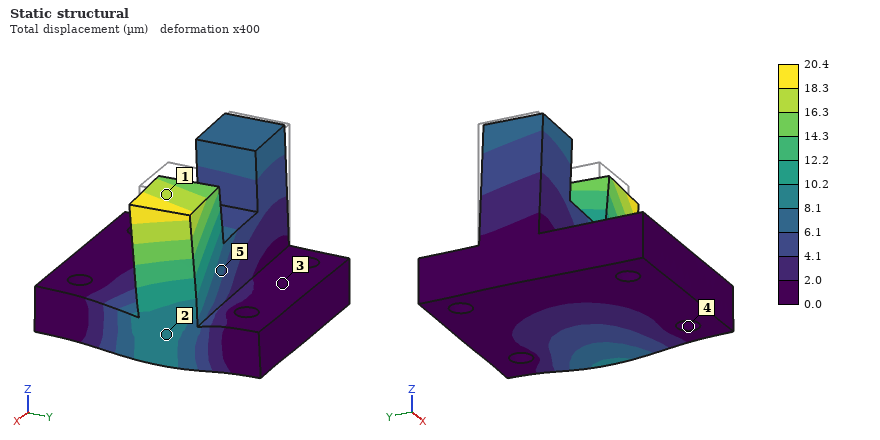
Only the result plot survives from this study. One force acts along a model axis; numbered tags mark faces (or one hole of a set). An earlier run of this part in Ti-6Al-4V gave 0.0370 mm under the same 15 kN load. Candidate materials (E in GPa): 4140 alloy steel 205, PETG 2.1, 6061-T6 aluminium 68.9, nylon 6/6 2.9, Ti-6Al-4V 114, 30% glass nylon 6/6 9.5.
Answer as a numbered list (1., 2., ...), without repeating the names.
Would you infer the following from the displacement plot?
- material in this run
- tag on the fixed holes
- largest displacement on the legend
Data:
1. 4140 alloy steel
2. 4
3. 20.4 µm
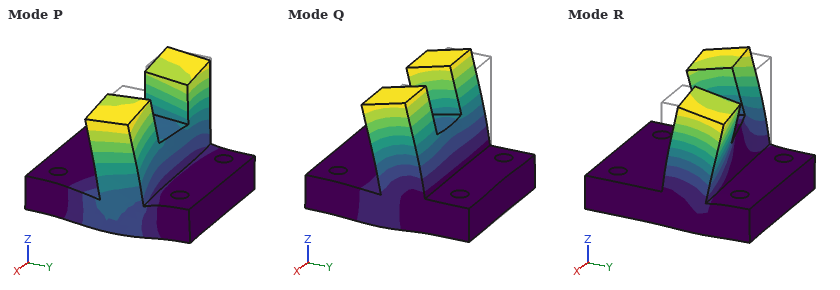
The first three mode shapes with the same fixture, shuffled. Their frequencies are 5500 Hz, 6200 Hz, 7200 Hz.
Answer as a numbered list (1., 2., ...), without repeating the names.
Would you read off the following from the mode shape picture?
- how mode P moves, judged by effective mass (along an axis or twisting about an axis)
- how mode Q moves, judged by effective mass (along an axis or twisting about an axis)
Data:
1. along X
2. along Y
